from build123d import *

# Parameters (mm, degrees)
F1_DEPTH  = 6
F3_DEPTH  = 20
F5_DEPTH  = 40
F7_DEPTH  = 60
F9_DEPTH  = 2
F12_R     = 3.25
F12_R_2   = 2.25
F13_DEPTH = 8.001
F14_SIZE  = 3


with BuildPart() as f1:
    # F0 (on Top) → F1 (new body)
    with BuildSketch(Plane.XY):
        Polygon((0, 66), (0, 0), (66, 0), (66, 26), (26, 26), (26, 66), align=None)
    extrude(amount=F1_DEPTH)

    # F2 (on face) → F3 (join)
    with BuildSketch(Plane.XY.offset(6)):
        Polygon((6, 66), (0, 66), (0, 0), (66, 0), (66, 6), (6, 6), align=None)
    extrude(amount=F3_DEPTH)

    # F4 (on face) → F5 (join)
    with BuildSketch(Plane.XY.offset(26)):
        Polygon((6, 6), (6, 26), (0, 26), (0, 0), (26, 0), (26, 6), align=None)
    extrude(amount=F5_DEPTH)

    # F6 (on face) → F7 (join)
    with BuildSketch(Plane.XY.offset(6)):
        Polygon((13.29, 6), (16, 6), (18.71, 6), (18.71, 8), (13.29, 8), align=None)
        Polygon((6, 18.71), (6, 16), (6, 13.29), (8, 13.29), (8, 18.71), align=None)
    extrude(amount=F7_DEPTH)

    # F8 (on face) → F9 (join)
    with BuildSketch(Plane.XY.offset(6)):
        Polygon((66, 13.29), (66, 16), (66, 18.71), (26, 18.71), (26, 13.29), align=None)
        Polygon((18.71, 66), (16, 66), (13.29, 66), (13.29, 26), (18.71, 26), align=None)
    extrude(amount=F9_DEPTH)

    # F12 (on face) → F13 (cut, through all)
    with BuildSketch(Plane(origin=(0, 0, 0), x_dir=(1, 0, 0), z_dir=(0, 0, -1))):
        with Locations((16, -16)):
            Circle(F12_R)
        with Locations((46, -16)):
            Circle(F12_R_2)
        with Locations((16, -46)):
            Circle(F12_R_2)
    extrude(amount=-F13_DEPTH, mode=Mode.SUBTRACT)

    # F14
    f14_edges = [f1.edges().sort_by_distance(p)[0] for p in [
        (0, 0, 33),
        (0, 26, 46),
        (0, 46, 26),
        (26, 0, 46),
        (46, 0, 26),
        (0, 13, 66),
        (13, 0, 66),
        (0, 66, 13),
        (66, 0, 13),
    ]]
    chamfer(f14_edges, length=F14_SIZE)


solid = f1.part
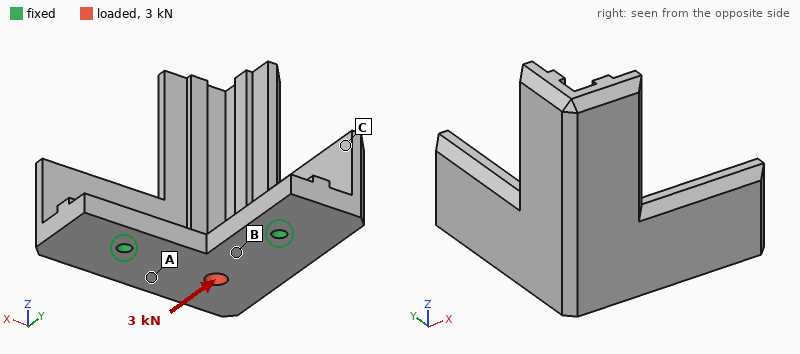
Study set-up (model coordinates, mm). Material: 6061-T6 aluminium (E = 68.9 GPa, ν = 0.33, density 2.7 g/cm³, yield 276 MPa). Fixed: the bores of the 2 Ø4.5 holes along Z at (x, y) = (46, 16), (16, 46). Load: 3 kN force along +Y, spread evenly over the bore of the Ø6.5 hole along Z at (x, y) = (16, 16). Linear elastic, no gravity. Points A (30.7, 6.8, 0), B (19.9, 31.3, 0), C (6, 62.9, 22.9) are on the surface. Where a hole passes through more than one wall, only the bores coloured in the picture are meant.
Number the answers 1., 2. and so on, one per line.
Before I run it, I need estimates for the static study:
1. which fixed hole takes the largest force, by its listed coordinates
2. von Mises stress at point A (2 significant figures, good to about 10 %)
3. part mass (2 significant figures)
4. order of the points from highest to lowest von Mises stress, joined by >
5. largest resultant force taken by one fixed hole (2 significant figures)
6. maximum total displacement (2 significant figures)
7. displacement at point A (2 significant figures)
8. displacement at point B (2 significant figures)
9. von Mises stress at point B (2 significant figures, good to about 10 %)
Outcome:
1. (16, 46)
2. 6.3 MPa
3. 120 g
4. B > A > C
5. 2.6 kN
6. 14 µm
7. 6.6 µm
8. 4.5 µm
9. 21 MPa
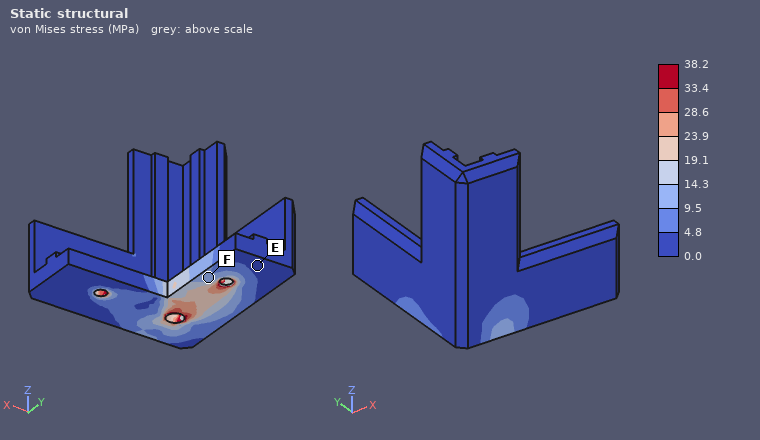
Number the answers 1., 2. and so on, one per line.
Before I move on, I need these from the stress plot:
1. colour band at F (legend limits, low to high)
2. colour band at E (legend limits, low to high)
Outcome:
1. 9.5 to 14.3 MPa
2. 0.0 to 4.8 MPa
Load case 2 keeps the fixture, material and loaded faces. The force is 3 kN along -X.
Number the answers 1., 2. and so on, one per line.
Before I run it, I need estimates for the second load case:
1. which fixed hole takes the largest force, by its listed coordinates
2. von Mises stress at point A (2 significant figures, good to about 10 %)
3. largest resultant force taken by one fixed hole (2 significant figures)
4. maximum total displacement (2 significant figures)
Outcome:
1. (46, 16)
2. 14 MPa
3. 2.6 kN
4. 14 µm
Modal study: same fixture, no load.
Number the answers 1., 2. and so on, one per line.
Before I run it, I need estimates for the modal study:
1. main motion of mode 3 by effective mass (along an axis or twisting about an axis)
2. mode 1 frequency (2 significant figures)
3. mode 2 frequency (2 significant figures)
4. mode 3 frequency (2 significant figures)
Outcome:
1. along Z
2. 1300 Hz
3. 3000 Hz
4. 5000 Hz
